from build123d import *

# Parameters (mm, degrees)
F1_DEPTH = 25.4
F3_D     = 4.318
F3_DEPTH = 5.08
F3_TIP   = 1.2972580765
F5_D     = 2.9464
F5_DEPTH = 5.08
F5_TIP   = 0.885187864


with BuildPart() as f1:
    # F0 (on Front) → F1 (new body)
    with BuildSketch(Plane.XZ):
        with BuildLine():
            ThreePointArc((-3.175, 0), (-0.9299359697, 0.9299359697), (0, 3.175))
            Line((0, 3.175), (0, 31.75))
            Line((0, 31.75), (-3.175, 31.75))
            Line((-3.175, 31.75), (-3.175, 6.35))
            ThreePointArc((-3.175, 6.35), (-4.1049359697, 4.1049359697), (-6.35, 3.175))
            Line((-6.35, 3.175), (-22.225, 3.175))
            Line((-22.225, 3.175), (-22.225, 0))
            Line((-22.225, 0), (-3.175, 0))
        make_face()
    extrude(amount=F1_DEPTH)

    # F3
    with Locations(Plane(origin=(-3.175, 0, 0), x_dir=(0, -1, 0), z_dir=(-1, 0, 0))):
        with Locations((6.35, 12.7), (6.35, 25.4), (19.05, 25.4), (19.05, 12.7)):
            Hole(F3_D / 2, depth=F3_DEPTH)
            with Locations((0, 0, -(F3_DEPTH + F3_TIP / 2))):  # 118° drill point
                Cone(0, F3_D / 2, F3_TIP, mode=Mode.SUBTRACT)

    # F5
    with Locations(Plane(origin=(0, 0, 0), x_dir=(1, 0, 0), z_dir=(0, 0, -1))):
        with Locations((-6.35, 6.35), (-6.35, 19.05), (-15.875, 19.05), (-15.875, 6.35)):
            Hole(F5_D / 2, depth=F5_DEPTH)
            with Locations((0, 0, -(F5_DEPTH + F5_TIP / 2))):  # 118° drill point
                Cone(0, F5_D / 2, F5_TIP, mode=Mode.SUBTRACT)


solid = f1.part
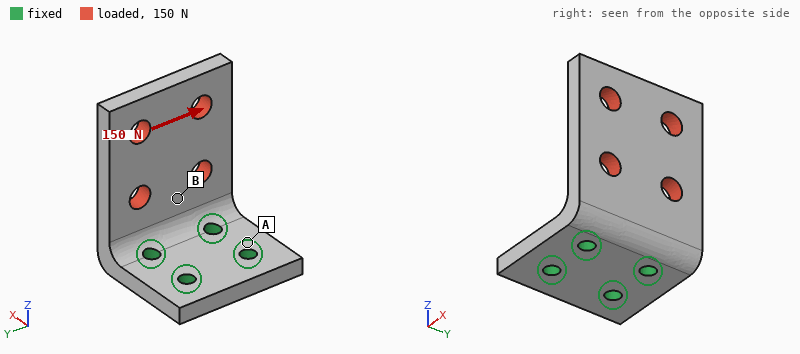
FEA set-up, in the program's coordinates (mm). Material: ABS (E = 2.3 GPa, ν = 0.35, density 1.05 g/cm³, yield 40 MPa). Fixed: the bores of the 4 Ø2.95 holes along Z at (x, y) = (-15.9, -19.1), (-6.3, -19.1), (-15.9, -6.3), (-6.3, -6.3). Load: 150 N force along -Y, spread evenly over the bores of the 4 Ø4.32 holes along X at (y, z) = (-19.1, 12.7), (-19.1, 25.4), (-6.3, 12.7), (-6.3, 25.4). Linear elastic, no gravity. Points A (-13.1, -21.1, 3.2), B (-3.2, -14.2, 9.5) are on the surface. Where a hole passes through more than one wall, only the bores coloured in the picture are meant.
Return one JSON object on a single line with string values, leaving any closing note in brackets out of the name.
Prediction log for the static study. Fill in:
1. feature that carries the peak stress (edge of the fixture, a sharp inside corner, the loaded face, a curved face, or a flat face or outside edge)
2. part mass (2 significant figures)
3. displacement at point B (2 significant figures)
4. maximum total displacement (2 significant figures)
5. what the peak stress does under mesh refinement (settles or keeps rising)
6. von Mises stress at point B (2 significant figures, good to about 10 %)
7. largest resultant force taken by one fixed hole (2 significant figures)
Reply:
{"feature that carries the peak stress": "edge of the fixture", "part mass": "4.0 g", "displacement at point B": "0.093 mm", "maximum total displacement": "0.41 mm", "what the peak stress does under mesh refinement": "keeps rising", "von Mises stress at point B": "7.5 MPa", "largest resultant force taken by one fixed hole": "190 N"}
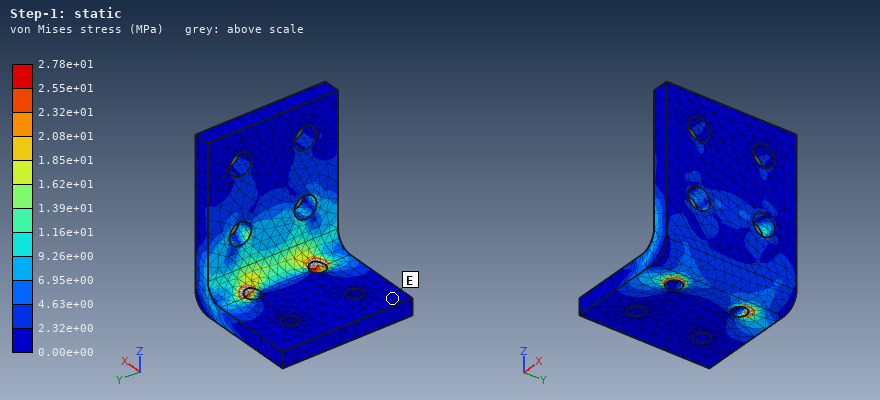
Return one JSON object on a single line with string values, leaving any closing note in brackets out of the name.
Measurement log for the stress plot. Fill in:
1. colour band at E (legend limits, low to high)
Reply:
{"colour band at E": "0.00e+00 to 2.32e+00 MPa"}
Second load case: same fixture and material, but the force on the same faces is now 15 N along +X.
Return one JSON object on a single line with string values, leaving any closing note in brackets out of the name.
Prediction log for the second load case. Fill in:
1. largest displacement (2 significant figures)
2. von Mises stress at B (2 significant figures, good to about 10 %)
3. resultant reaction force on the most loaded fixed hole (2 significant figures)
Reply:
{"largest displacement": "0.43 mm", "von Mises stress at B": "3.7 MPa", "resultant reaction force on the most loaded fixed hole": "8.7 N"}
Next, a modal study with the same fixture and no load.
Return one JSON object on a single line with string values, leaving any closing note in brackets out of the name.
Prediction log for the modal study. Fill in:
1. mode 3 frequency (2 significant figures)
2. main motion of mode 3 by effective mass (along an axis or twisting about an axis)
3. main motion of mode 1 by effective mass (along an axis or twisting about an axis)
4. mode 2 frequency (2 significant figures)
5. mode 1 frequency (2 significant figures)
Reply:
{"mode 3 frequency": "2900 Hz", "main motion of mode 3 by effective mass": "along Y", "main motion of mode 1 by effective mass": "along X", "mode 2 frequency": "2100 Hz", "mode 1 frequency": "820 Hz"}
